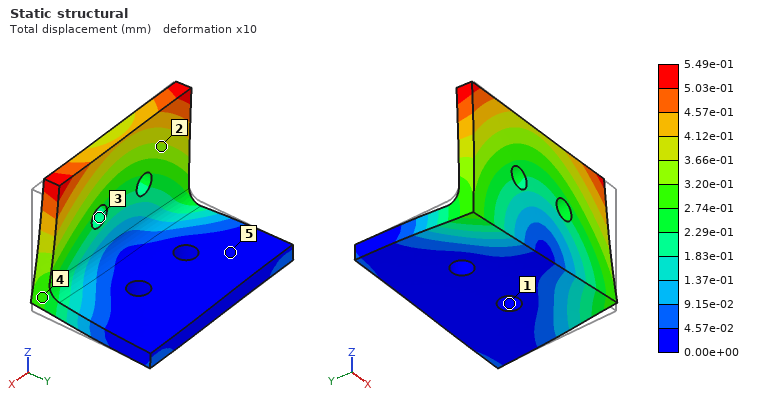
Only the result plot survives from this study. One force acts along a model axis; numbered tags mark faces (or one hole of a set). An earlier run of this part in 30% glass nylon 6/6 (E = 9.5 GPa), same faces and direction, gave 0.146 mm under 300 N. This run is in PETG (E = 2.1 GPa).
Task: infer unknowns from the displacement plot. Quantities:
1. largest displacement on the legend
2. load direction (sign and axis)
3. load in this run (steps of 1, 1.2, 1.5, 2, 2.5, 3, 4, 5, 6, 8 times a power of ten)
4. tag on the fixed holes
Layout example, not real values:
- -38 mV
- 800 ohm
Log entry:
- 5.49e-01 mm
- -X
- 250 N
- 1
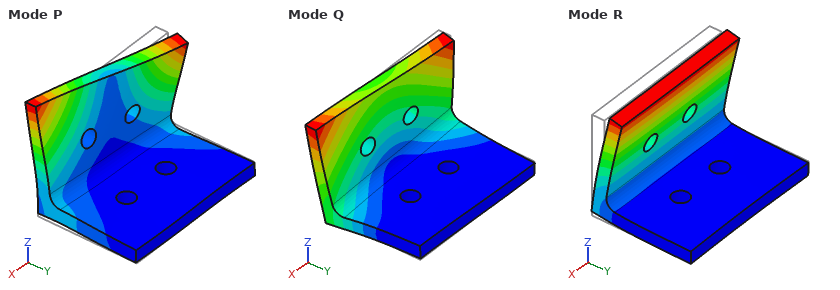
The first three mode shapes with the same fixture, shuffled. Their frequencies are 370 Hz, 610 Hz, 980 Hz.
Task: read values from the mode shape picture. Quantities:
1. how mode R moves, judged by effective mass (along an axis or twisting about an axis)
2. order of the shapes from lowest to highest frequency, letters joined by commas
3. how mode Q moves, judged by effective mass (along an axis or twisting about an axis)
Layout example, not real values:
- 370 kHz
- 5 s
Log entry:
- along Y
- R, Q, P
- along X
